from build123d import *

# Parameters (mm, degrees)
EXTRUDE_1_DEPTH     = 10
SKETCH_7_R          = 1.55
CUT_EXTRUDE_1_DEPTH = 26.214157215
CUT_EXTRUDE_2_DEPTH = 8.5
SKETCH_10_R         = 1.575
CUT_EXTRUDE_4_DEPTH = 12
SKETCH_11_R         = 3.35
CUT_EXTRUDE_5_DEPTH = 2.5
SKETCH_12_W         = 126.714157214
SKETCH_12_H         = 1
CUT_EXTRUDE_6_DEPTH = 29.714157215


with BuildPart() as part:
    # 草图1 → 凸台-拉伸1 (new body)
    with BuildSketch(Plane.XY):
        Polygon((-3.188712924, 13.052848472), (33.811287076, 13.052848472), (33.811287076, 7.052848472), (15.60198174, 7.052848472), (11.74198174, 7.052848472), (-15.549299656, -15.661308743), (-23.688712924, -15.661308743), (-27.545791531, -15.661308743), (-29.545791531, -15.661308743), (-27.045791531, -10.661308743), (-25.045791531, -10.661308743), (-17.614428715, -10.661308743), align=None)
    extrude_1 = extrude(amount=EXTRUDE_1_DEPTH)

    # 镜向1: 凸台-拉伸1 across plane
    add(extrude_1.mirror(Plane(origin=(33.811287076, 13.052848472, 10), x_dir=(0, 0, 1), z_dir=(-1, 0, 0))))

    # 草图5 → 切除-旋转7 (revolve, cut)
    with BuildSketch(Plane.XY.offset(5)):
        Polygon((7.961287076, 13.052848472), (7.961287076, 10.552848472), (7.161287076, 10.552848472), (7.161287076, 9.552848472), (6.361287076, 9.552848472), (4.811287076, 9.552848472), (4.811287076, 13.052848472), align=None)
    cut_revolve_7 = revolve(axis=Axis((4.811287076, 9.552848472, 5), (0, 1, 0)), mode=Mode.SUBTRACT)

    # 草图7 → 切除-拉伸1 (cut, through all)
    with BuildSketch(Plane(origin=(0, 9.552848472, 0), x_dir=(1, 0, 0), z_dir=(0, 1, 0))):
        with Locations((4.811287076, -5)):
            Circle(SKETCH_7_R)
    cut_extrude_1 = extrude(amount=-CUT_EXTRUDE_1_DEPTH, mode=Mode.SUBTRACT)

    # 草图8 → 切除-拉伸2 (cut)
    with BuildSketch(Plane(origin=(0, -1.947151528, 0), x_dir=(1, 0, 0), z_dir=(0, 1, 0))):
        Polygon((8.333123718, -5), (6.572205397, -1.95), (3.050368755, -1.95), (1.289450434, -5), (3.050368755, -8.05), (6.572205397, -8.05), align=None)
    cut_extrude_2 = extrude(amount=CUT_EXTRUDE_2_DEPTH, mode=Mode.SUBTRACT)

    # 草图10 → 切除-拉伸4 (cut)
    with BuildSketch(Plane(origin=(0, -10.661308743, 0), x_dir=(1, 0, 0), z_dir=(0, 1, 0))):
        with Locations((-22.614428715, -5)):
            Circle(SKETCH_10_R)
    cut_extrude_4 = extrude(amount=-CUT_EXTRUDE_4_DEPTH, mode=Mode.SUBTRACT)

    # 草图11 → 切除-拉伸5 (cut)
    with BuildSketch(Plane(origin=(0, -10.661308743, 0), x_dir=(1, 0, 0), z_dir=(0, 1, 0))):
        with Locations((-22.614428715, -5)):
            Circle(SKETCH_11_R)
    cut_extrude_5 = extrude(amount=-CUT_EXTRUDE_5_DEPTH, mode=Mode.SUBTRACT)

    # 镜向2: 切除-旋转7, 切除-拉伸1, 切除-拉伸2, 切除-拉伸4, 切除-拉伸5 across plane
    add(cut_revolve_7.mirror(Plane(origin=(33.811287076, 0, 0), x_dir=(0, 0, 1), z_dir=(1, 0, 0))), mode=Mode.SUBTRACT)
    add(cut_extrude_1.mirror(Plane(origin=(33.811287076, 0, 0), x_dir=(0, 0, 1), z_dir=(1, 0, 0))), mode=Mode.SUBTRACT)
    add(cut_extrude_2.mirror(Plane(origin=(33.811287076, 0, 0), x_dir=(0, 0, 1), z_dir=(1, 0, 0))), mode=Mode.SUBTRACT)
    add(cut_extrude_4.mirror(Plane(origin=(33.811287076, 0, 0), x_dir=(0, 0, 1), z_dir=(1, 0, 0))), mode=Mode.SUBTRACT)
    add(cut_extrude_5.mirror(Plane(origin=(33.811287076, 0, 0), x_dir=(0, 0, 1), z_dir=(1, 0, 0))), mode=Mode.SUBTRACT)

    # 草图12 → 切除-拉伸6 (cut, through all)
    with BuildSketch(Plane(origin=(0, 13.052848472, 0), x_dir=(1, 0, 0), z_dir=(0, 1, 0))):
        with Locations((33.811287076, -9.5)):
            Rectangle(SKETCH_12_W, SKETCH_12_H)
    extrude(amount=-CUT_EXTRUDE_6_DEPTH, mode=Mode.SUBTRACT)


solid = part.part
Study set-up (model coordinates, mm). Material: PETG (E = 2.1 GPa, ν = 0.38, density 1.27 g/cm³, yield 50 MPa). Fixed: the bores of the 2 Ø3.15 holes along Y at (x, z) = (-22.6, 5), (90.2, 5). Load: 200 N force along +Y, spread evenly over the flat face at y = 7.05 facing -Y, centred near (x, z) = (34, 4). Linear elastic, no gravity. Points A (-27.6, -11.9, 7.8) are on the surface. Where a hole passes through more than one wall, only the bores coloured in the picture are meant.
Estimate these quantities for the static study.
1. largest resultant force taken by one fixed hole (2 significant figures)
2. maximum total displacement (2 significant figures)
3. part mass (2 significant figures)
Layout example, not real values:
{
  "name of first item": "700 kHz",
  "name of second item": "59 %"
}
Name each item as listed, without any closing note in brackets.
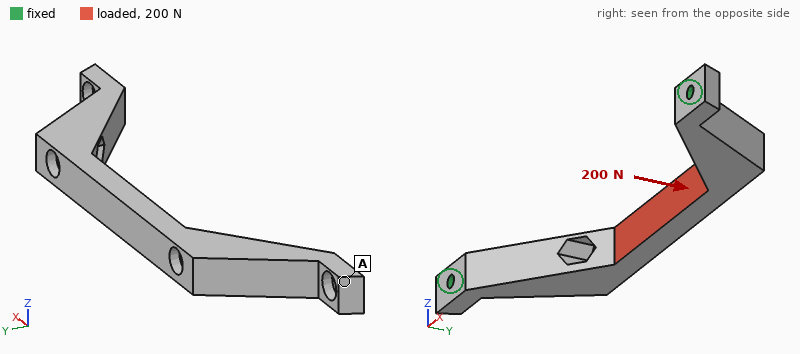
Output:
{
  "largest resultant force taken by one fixed hole": "180 N",
  "maximum total displacement": "0.63 mm",
  "part mass": "12 g"
}
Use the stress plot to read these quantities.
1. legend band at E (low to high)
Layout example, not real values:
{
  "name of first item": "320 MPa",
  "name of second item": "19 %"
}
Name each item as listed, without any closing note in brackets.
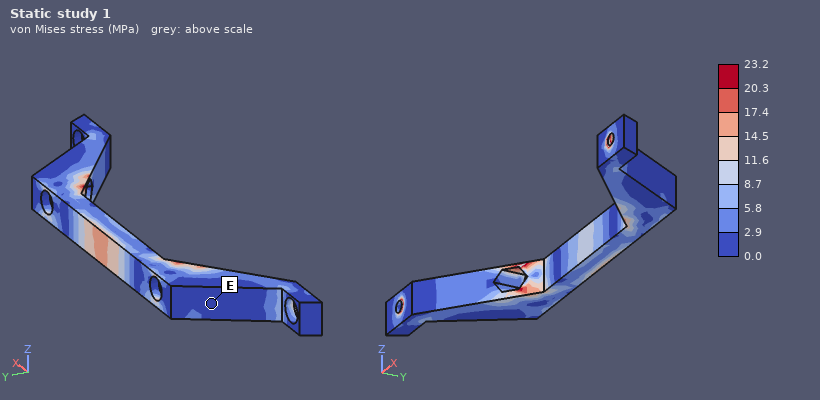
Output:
{
  "legend band at E": "0.0 to 2.9 MPa"
}
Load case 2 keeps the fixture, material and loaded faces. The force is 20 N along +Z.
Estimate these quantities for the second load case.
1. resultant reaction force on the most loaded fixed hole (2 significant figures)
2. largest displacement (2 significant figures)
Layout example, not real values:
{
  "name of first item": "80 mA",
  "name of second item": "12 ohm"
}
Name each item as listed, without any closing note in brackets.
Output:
{
  "resultant reaction force on the most loaded fixed hole": "10 N",
  "largest displacement": "0.62 mm"
}
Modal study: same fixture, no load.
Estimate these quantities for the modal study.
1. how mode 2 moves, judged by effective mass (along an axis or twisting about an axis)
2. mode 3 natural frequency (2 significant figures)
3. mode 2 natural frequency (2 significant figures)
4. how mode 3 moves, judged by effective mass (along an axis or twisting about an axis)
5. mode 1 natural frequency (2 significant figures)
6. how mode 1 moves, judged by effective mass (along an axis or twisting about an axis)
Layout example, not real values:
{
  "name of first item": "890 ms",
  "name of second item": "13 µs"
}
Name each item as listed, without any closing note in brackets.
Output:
{
  "how mode 2 moves, judged by effective mass": "along X",
  "mode 3 natural frequency": "960 Hz",
  "mode 2 natural frequency": "890 Hz",
  "how mode 3 moves, judged by effective mass": "twisting about Y",
  "mode 1 natural frequency": "380 Hz",
  "how mode 1 moves, judged by effective mass": "along Z"
}
